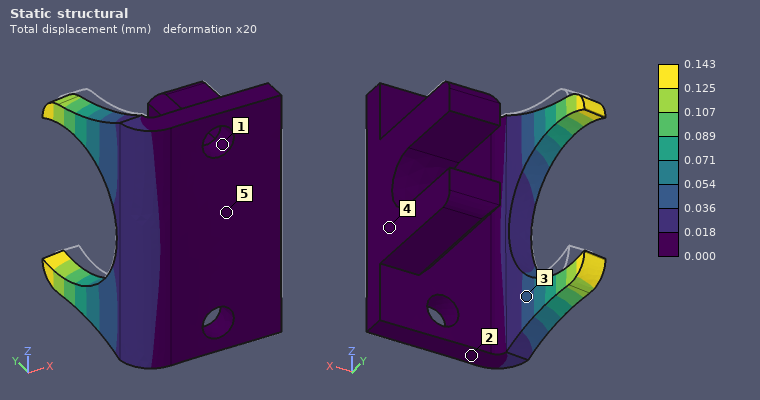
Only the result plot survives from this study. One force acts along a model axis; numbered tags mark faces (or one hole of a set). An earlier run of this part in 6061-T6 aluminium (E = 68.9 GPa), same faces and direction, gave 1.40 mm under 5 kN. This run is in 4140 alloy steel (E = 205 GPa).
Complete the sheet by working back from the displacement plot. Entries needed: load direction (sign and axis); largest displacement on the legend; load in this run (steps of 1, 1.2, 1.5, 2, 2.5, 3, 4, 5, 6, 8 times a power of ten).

-X
0.143 mm
1.5 kN
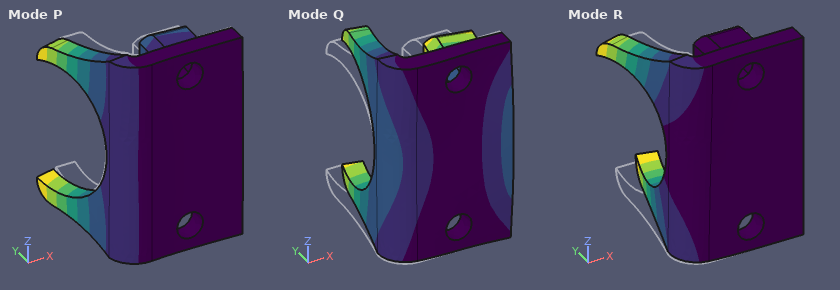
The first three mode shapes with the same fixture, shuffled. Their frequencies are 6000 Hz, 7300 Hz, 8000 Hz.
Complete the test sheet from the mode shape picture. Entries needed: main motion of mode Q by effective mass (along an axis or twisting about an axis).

along X
